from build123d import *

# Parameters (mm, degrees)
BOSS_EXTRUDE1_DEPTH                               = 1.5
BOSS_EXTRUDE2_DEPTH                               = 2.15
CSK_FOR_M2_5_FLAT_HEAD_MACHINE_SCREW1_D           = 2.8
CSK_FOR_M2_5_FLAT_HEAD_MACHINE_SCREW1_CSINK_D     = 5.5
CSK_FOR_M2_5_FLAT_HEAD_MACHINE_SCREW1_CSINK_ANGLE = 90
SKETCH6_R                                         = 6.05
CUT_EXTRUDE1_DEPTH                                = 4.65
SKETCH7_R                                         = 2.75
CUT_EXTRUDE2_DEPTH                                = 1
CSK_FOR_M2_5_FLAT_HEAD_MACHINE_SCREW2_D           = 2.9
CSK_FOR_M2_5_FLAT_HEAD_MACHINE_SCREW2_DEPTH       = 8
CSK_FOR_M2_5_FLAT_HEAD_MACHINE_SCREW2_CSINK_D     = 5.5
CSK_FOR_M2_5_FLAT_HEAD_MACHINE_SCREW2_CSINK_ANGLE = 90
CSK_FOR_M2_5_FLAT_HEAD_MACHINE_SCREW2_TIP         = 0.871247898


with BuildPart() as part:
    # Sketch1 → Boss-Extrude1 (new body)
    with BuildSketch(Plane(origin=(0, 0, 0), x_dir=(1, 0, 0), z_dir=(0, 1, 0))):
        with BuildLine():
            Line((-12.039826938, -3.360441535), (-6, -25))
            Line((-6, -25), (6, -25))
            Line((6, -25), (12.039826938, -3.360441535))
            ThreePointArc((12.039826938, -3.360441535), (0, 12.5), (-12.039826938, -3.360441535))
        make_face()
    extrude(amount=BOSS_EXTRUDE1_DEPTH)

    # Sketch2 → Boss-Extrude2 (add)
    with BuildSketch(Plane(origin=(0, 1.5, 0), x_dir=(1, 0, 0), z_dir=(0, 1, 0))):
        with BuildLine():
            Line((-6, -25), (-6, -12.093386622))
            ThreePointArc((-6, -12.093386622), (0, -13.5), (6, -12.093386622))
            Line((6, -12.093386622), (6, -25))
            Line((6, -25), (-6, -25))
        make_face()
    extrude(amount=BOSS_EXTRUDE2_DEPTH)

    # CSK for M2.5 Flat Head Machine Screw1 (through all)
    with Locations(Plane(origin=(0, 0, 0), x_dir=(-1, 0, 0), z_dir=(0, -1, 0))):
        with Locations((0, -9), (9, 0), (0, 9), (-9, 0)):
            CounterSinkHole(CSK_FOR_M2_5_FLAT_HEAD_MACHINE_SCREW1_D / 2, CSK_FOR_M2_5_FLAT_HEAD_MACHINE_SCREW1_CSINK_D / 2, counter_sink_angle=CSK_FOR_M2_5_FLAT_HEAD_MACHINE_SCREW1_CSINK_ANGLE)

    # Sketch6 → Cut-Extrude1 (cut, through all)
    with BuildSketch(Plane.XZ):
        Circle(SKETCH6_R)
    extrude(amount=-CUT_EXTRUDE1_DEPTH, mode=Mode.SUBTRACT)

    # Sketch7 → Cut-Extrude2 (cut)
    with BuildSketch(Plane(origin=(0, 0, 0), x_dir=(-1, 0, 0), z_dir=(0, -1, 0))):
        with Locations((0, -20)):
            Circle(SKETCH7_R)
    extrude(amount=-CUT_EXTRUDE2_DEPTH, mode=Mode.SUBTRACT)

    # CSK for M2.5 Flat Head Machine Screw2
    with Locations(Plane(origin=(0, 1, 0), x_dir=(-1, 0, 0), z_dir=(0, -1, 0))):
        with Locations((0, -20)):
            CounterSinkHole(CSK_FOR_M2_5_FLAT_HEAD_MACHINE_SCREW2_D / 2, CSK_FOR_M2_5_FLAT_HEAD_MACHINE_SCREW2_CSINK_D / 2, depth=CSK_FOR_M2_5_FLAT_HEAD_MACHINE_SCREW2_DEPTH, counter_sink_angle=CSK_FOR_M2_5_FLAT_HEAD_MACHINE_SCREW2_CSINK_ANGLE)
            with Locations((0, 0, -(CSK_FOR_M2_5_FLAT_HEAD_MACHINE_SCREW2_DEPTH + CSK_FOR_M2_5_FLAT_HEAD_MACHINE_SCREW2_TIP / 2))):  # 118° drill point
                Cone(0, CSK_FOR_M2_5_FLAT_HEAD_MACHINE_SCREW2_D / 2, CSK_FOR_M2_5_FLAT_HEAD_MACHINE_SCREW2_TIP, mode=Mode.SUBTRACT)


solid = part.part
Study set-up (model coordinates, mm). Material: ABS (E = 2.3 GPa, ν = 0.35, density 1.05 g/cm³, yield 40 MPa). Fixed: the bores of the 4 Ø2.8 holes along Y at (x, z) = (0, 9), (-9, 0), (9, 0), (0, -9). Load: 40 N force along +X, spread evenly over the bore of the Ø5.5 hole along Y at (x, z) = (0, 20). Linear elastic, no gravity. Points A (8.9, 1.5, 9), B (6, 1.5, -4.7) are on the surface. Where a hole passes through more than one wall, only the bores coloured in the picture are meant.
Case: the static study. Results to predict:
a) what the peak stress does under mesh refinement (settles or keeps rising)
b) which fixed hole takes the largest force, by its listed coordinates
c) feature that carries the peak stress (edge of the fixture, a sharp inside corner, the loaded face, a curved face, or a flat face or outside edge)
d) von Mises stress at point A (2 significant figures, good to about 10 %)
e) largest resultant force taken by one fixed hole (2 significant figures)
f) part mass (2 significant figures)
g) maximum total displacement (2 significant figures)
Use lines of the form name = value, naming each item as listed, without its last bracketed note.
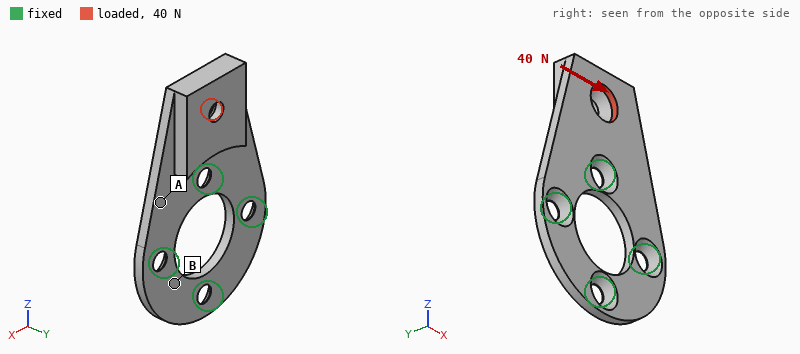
what the peak stress does under mesh refinement = keeps rising
which fixed hole takes the largest force, by its listed coordinates = (0, 9)
feature that carries the peak stress = edge of the fixture
von Mises stress at point A = 3.8 MPa
largest resultant force taken by one fixed hole = 35 N
part mass = 1.1 g
maximum total displacement = 0.12 mm
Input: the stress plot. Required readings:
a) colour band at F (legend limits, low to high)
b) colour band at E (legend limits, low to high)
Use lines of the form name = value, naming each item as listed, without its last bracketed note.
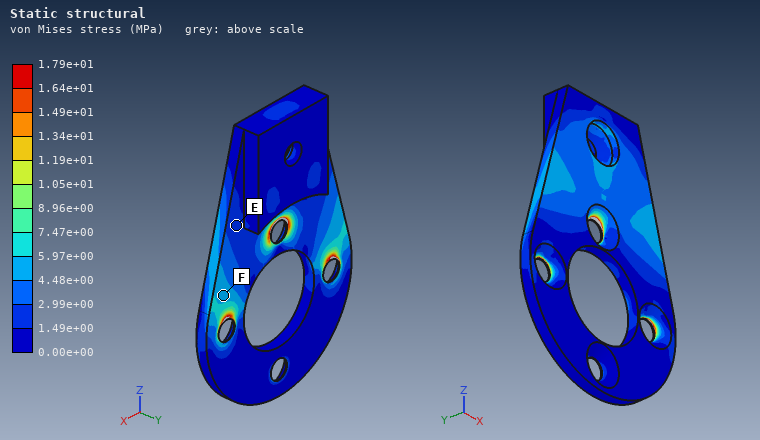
colour band at F = 4.48e+00 to 5.97e+00 MPa
colour band at E = 1.49e+00 to 2.99e+00 MPa
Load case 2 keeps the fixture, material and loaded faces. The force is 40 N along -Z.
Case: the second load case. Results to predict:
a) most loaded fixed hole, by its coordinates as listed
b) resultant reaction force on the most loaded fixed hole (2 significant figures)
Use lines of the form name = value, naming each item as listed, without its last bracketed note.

most loaded fixed hole, by its coordinates as listed = (0, 9)
resultant reaction force on the most loaded fixed hole = 15 N
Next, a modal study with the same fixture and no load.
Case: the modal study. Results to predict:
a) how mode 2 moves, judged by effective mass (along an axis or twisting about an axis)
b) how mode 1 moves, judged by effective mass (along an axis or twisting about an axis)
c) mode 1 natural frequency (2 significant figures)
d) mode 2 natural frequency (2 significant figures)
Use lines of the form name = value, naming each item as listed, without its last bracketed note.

how mode 2 moves, judged by effective mass = twisting about Z
how mode 1 moves, judged by effective mass = along Y
mode 1 natural frequency = 950 Hz
mode 2 natural frequency = 2200 Hz
